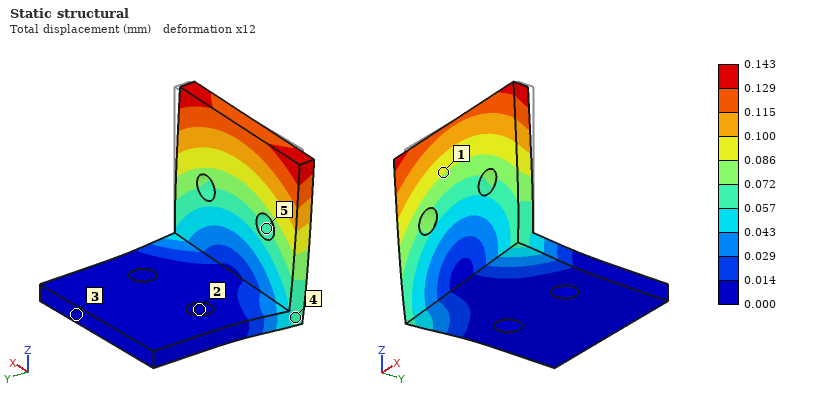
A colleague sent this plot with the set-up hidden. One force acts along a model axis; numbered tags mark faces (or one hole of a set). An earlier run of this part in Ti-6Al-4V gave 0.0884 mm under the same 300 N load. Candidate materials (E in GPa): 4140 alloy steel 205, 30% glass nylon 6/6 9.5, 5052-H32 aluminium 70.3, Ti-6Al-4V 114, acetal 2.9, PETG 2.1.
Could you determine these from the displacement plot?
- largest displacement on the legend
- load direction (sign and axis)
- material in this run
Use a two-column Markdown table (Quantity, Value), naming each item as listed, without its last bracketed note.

| Quantity | Value |
|---|---|
| largest displacement on the legend | 0.143 mm |
| load direction | -X |
| material in this run | 5052-H32 aluminium |
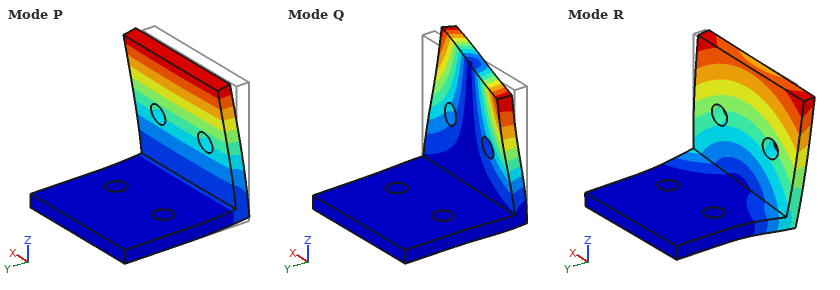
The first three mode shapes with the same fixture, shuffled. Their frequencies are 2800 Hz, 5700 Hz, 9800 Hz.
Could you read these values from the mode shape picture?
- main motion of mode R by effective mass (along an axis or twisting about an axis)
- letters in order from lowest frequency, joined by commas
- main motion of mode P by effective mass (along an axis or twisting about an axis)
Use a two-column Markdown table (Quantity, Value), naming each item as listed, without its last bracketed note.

| Quantity | Value |
|---|---|
| main motion of mode R by effective mass | along X |
| letters in order from lowest frequency, joined by commas | P, R, Q |
| main motion of mode P by effective mass | along Y |
